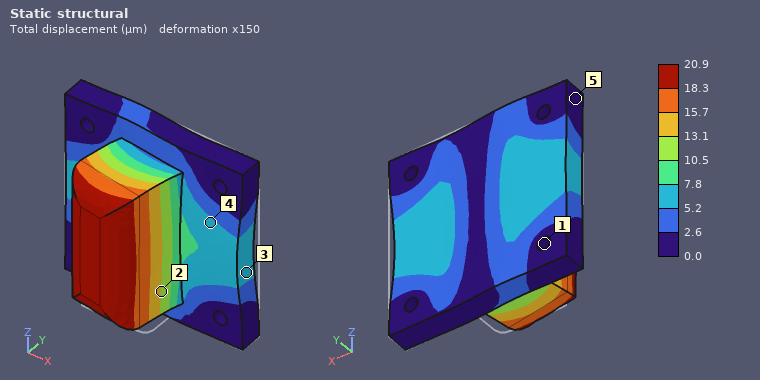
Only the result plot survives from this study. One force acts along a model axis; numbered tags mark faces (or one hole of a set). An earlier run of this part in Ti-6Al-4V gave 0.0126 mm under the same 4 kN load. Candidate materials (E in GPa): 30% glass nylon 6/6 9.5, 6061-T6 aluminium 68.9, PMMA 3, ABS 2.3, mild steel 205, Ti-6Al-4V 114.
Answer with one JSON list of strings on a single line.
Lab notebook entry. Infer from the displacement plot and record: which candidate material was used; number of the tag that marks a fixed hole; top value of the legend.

["6061-T6 aluminium", "1", "20.9 µm"]
